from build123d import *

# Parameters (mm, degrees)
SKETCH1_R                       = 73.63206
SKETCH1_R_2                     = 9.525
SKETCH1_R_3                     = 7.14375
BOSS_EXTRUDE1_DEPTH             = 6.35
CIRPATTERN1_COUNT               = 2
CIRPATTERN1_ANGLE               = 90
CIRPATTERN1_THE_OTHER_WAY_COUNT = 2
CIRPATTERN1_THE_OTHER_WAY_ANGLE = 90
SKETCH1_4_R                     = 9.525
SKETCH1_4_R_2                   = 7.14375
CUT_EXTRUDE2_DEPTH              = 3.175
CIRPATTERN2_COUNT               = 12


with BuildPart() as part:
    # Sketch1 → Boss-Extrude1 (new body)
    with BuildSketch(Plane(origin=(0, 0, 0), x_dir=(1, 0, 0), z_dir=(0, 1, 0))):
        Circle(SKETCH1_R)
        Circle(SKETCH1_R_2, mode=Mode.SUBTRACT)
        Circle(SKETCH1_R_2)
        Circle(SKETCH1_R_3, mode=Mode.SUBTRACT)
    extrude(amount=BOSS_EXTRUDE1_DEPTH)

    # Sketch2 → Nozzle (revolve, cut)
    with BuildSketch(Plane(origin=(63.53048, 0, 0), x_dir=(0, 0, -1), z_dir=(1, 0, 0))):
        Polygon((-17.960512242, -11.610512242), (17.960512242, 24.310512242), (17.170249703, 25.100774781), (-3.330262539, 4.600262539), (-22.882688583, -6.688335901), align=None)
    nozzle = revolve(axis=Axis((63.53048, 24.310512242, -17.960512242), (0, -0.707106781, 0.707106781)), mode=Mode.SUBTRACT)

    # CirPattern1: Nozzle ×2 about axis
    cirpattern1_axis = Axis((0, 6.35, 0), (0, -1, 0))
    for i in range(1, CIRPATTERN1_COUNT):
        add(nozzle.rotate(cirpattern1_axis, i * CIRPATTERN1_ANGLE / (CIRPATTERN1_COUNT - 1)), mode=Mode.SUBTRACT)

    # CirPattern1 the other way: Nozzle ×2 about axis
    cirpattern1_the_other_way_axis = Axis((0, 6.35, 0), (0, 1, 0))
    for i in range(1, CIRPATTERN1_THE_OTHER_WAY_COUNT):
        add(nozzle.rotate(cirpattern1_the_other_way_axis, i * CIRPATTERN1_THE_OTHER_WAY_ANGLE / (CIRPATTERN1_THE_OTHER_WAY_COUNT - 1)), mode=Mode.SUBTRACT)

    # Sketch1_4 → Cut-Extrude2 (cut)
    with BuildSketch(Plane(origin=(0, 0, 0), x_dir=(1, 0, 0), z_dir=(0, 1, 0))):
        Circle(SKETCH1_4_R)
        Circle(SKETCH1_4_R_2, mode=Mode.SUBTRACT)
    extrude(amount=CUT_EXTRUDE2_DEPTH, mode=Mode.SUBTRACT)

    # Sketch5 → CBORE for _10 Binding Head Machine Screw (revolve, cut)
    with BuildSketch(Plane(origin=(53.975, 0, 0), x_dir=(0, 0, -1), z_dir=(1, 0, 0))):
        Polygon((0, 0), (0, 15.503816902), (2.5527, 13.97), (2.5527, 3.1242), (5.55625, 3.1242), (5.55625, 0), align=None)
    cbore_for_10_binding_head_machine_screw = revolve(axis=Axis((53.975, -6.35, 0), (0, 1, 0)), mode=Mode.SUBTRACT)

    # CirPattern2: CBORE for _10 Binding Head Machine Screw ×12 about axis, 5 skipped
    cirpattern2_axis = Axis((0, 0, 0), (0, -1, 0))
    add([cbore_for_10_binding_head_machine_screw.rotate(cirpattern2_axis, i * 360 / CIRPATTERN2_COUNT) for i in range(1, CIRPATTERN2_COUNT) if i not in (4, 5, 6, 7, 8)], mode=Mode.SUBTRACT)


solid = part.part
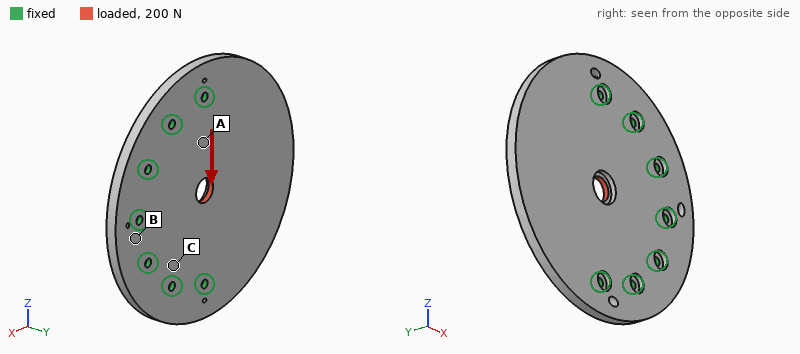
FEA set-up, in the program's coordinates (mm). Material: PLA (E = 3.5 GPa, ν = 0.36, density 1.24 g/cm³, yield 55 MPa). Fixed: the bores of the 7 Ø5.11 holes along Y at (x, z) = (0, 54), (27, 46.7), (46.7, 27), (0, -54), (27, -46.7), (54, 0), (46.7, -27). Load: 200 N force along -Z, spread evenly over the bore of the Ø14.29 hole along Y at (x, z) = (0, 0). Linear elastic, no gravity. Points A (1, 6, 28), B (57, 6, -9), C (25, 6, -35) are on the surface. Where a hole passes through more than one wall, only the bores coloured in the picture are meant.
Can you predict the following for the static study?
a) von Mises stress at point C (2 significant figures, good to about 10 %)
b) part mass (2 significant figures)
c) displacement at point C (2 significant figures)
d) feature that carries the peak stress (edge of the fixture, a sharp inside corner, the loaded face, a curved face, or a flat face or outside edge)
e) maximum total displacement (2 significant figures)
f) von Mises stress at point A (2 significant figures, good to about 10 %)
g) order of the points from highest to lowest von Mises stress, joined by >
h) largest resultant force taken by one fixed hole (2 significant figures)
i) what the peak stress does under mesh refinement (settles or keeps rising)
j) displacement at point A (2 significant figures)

0.38 MPa
130 g
2.1 µm
edge of the fixture
10 µm
0.58 MPa
A > C > B
56 N
keeps rising
6.3 µm
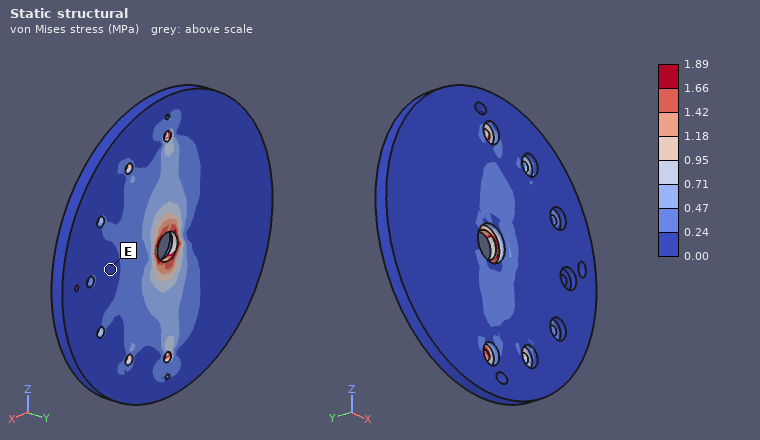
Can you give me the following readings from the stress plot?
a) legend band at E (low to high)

0.00 to 0.24 MPa
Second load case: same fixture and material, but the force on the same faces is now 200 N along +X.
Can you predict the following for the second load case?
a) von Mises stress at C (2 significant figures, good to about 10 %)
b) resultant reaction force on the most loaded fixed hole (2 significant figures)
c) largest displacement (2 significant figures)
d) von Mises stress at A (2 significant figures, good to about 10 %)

0.26 MPa
36 N
30 µm
0.32 MPa
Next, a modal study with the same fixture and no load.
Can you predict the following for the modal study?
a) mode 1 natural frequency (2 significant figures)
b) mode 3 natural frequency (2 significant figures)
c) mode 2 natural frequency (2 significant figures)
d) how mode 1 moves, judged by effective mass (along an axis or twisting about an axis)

280 Hz
1100 Hz
720 Hz
along Y
